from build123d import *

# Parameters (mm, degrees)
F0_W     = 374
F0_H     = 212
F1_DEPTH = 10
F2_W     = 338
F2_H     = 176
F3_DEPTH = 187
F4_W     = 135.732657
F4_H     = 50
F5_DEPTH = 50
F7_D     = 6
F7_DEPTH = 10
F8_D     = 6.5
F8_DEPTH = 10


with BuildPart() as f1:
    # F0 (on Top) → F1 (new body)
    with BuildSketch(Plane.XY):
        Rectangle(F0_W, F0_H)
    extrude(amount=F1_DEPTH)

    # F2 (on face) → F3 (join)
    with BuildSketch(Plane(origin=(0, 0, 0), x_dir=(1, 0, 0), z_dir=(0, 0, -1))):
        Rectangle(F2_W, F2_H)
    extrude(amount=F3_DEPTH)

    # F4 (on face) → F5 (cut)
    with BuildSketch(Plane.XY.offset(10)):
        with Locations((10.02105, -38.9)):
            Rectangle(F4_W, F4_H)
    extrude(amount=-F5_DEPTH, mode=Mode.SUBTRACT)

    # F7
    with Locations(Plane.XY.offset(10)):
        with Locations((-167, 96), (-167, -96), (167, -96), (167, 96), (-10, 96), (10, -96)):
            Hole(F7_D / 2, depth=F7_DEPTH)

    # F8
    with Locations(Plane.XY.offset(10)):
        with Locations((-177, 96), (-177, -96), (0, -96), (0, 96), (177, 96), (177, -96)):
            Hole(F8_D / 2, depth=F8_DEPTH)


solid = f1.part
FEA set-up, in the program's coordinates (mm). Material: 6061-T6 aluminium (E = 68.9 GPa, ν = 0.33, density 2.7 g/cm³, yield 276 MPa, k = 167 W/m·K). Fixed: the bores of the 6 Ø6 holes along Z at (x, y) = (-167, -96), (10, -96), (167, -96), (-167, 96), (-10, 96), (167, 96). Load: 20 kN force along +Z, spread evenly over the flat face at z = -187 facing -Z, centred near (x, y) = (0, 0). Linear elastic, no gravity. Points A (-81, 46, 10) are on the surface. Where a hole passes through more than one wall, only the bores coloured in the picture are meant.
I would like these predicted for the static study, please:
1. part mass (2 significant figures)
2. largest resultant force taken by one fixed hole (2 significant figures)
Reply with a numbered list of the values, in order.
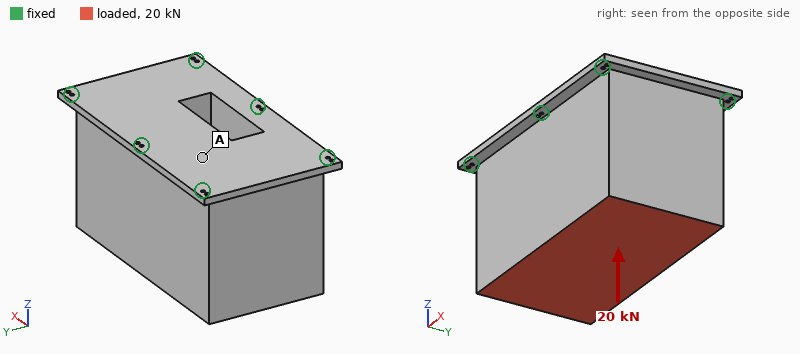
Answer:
1. 31 kg
2. 4.6 kN
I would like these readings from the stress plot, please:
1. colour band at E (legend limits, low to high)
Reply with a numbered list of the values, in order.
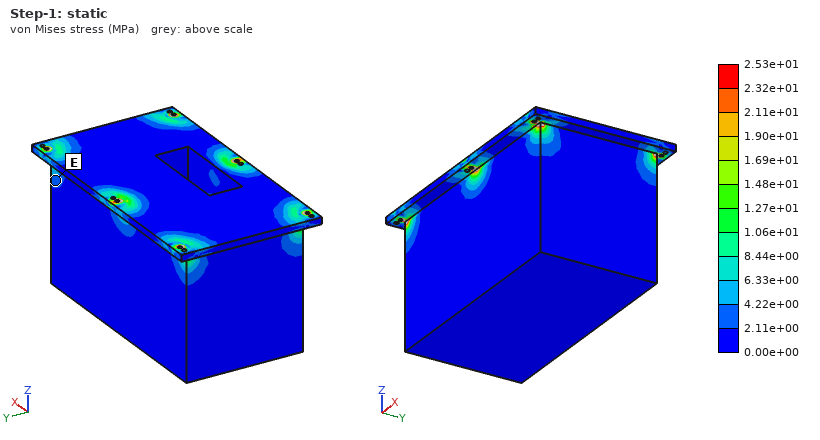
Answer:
1. 2.11e+00 to 4.22e+00 MPa
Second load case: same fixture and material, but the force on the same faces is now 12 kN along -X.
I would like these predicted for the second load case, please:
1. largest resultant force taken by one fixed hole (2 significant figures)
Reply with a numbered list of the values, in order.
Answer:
1. 4.5 kN
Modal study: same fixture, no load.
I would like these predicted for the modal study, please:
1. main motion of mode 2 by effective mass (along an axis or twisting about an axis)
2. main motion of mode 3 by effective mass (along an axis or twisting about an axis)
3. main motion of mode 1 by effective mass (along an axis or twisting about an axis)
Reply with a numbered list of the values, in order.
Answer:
1. along X
2. along Z
3. along Y
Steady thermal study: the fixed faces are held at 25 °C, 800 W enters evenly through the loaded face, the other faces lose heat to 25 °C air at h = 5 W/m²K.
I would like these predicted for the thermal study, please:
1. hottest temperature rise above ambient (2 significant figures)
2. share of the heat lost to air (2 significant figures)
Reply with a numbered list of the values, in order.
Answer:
1. 60 K
2. 9.5 %
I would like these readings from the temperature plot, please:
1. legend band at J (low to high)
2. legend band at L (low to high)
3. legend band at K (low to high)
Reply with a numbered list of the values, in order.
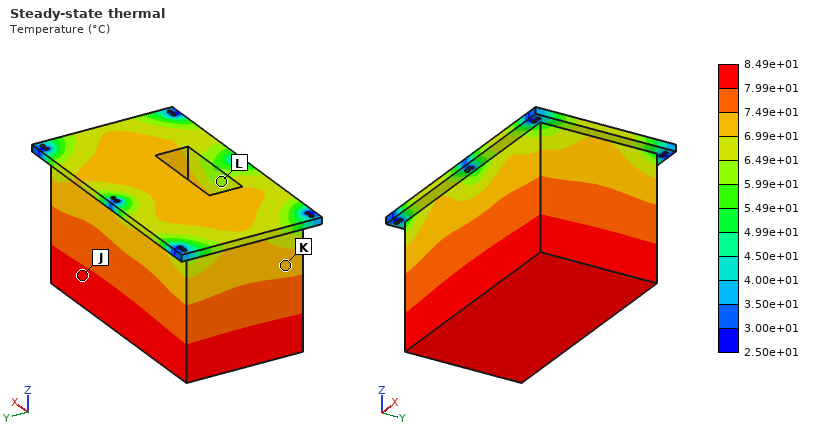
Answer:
1. 7.99e+01 to 8.49e+01 °C
2. 5.99e+01 to 6.49e+01 °C
3. 6.99e+01 to 7.49e+01 °C
